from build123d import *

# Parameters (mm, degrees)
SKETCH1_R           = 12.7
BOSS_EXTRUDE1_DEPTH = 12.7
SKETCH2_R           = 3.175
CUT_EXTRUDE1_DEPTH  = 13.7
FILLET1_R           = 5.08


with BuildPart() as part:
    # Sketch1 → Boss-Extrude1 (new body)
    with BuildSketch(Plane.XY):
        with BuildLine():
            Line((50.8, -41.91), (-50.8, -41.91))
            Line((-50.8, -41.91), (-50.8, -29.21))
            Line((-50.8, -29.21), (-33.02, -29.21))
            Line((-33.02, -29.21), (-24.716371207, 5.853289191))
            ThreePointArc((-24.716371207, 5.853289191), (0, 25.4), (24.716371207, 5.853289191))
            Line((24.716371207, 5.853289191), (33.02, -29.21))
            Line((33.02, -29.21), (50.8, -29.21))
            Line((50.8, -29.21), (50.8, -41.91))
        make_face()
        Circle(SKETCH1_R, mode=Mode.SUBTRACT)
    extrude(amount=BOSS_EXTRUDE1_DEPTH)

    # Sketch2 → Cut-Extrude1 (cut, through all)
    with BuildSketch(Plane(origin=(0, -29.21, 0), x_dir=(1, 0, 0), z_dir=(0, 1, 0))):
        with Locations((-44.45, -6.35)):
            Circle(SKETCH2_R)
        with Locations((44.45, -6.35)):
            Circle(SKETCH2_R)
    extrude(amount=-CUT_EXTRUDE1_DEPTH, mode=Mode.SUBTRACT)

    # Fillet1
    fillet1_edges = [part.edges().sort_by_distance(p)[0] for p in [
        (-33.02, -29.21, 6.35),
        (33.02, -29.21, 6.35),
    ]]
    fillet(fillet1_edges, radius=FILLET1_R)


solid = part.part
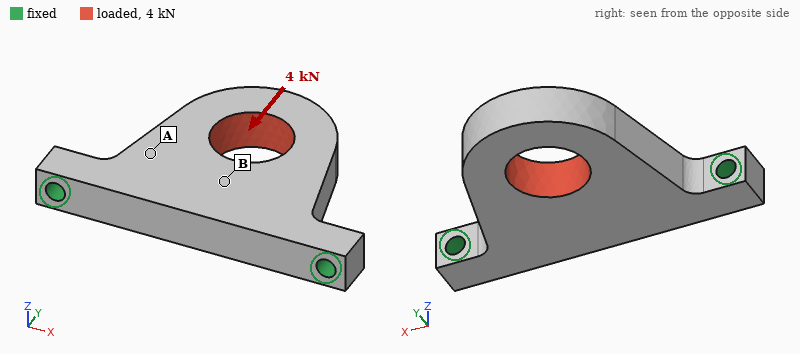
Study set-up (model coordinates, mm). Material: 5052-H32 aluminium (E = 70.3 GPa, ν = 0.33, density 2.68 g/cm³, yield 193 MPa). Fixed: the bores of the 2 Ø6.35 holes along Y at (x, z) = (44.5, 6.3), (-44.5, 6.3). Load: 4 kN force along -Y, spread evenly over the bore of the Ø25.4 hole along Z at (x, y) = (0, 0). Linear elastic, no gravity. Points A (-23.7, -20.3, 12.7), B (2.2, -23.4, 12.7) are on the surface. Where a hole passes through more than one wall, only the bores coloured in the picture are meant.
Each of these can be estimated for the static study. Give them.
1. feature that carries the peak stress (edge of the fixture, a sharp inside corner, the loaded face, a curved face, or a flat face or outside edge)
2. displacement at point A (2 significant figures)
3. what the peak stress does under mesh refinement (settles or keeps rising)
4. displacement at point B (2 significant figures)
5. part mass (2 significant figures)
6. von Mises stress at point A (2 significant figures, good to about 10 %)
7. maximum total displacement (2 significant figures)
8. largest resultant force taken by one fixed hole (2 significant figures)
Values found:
edge of the fixture
13 µm
keeps rising
17 µm
120 g
12 MPa
18 µm
2.3 kN
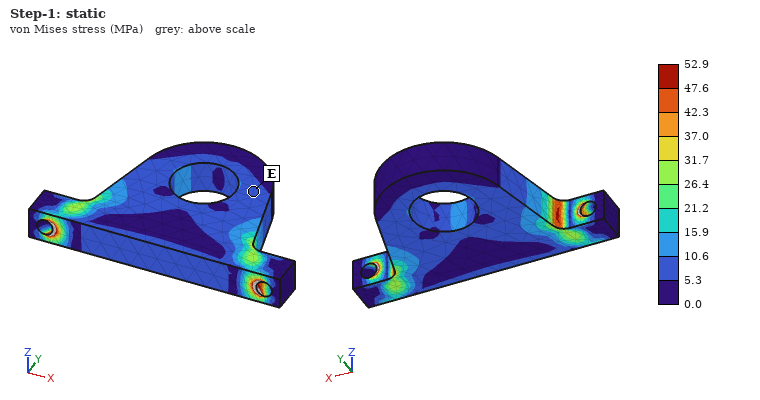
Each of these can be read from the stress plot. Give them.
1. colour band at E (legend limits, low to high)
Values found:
5.3 to 10.6 MPa
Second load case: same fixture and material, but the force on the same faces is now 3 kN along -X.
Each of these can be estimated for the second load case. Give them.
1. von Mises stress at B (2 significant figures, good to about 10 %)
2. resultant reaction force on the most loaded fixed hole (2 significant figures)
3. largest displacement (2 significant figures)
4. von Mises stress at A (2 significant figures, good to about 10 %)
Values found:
8.1 MPa
2.1 kN
27 µm
9.0 MPa
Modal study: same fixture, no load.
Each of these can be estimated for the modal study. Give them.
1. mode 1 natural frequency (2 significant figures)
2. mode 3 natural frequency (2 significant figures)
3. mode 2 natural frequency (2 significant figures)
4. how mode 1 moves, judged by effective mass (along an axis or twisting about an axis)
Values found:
1800 Hz
6900 Hz
6700 Hz
along Z
